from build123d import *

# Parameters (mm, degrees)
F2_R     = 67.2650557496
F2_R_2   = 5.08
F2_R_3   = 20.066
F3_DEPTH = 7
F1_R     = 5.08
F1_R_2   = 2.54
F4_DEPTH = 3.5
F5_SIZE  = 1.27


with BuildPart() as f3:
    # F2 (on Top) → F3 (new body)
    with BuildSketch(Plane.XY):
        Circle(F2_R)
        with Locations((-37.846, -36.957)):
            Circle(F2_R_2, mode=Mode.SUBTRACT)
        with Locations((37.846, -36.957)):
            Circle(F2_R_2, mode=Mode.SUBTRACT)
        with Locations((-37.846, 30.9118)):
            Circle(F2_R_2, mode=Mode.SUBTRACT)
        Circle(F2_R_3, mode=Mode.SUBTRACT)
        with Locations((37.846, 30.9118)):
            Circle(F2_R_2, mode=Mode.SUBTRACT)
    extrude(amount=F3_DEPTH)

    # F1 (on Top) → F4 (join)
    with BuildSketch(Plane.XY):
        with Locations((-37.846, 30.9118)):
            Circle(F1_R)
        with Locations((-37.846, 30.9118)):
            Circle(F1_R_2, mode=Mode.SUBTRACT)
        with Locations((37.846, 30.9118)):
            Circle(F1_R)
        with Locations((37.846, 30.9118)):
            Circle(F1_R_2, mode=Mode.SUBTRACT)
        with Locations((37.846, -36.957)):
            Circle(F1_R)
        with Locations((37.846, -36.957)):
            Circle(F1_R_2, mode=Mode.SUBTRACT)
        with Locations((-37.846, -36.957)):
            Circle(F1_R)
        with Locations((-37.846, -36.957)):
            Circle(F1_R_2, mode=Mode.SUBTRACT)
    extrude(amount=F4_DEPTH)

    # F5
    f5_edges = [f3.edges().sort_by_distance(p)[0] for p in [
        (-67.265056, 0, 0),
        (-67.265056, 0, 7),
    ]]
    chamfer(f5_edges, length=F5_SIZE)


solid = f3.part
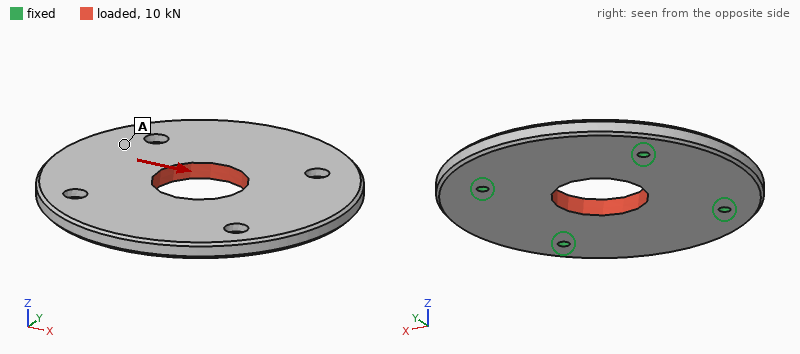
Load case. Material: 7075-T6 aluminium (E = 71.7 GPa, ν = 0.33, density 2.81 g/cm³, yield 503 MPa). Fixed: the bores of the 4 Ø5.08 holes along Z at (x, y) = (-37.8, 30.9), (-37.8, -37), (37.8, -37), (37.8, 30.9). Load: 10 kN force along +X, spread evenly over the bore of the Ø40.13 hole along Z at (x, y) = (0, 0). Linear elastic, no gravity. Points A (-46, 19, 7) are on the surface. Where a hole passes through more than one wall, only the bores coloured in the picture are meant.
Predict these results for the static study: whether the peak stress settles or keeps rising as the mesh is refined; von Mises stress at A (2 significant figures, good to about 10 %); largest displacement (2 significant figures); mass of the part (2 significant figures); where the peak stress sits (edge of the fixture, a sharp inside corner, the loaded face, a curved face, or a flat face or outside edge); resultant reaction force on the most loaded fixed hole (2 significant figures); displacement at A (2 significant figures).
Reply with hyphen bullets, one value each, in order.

- keeps rising
- 6.9 MPa
- 14 µm
- 250 g
- edge of the fixture
- 2.7 kN
- 8.0 µm
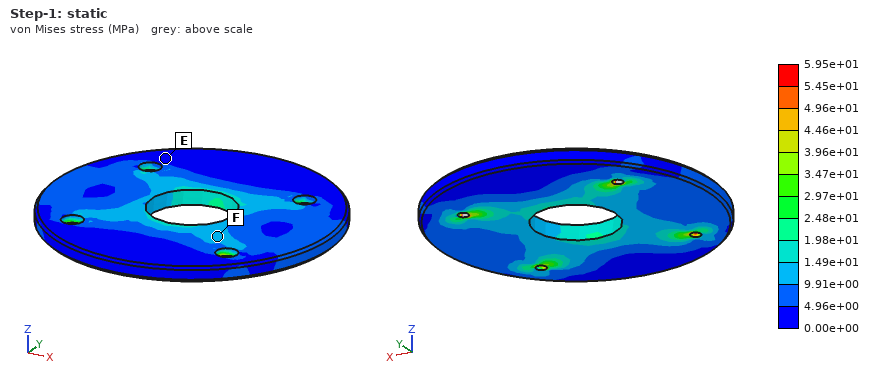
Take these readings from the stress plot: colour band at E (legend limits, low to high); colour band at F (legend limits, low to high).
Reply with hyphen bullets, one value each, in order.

- 0.00e+00 to 4.96e+00 MPa
- 9.91e+00 to 1.49e+01 MPa
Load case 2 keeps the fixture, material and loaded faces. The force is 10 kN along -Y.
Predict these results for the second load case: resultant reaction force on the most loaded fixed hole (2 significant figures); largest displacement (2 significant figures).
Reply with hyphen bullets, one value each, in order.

- 2.6 kN
- 17 µm
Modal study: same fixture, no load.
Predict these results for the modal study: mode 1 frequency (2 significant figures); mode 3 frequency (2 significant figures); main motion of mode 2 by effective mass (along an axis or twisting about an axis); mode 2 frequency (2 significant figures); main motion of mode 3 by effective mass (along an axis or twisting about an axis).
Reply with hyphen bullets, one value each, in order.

- 2700 Hz
- 4100 Hz
- twisting about X
- 3400 Hz
- twisting about Y
